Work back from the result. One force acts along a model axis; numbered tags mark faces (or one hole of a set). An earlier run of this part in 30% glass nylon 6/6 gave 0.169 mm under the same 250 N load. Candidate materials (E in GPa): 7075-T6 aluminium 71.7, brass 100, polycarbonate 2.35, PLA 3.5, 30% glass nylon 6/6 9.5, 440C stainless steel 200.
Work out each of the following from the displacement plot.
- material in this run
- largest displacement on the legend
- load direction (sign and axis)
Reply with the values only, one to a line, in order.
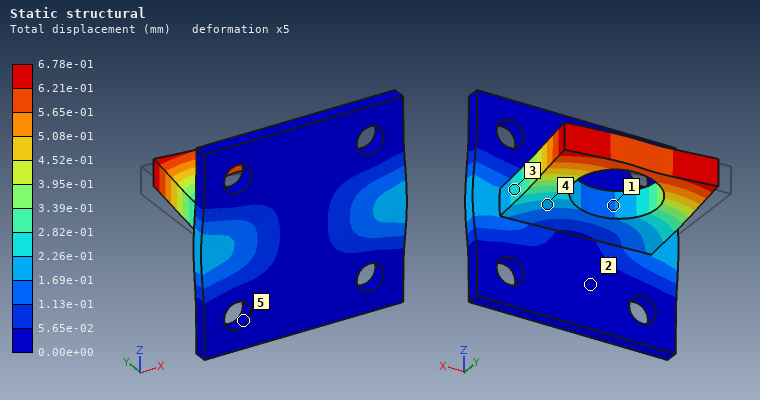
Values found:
polycarbonate
6.78e-01 mm
+X
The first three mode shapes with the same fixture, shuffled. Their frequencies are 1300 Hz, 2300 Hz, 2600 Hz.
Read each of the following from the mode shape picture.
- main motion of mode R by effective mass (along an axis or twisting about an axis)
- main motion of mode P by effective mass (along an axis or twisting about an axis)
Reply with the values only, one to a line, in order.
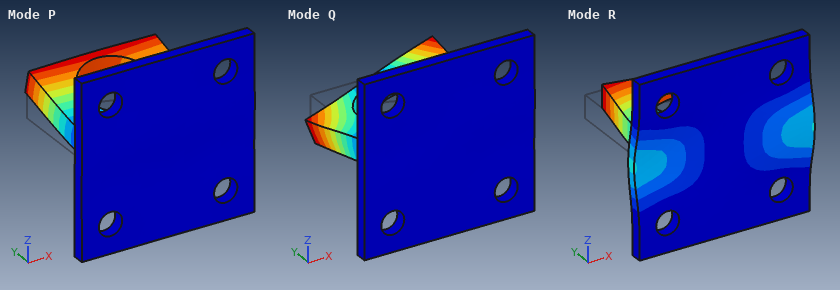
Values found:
along X
along Z
